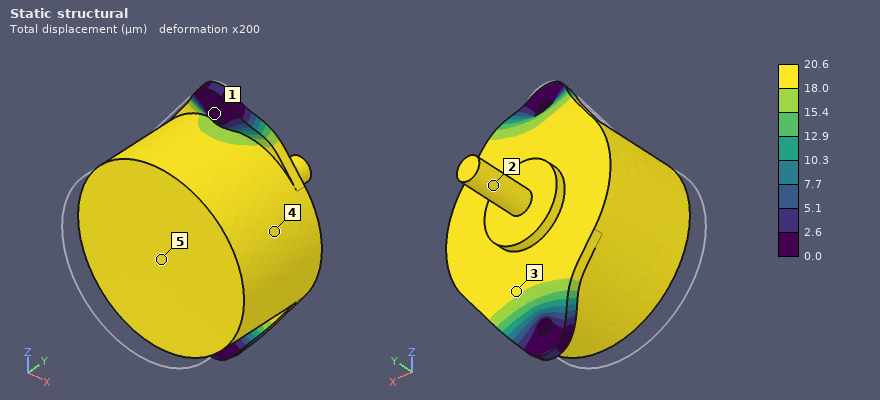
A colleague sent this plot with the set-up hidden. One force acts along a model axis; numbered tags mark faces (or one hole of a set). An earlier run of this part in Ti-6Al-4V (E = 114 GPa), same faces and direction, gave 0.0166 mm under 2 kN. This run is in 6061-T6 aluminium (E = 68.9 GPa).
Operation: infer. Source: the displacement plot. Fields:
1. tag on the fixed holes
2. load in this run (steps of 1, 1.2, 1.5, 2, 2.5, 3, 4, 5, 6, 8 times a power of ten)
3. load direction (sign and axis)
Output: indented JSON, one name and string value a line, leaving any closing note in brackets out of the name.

{
  "tag on the fixed holes": "1",
  "load in this run": "1.5 kN",
  "load direction": "+Y"
}
